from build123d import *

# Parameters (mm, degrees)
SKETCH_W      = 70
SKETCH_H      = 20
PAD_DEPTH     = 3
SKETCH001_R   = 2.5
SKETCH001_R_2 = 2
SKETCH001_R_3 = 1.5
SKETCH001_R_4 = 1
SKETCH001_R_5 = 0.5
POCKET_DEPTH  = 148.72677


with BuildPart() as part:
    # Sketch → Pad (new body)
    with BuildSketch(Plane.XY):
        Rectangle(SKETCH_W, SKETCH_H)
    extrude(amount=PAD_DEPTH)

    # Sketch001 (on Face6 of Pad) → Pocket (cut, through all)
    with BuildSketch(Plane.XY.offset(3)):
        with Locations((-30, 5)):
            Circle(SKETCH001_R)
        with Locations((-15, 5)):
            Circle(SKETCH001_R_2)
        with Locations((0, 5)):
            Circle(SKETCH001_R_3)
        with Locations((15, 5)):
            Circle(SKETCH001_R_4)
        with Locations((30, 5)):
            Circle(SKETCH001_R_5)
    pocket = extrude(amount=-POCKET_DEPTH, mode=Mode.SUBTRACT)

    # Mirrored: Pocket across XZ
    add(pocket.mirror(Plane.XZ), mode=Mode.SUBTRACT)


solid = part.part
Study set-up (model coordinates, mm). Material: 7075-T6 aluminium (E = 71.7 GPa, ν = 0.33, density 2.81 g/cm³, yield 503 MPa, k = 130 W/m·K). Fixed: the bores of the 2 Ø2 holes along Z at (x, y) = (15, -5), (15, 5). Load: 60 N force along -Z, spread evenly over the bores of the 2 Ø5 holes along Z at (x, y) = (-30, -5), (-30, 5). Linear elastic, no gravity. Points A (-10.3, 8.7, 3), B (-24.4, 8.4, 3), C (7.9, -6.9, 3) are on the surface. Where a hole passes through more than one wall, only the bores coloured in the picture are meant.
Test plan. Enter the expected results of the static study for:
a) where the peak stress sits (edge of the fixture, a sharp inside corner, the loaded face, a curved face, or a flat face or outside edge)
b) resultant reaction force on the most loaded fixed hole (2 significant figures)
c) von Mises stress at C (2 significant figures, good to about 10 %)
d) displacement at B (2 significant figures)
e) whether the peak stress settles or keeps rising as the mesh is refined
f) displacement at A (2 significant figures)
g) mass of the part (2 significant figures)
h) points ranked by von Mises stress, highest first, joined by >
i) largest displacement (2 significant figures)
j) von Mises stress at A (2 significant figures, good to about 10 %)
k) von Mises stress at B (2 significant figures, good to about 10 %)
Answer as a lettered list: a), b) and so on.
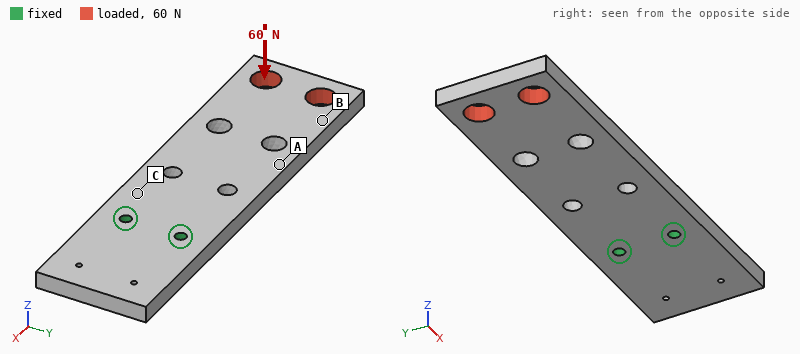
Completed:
a) edge of the fixture
b) 30 N
c) 74 MPa
d) 0.49 mm
e) keeps rising
f) 0.23 mm
g) 11 g
h) C > A > B
i) 0.71 mm
j) 43 MPa
k) 12 MPa
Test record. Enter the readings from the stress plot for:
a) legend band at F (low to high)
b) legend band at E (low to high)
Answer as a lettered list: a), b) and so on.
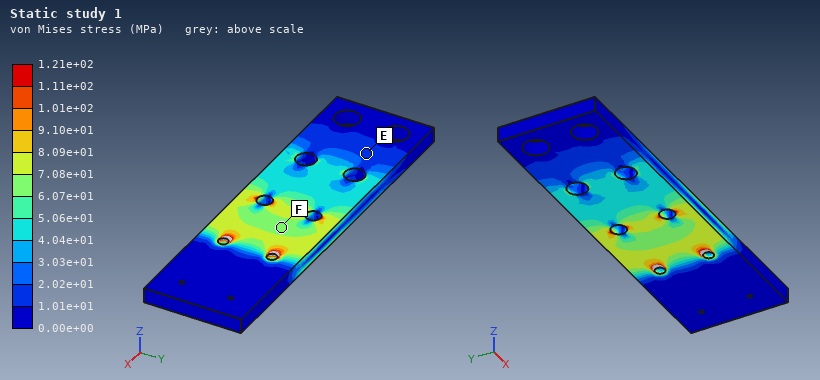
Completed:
a) 6.07e+01 to 7.08e+01 MPa
b) 1.01e+01 to 2.02e+01 MPa
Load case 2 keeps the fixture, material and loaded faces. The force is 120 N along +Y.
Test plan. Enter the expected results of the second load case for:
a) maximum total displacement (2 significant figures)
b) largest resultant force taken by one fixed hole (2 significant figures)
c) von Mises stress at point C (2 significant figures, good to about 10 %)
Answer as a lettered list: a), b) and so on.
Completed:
a) 45 µm
b) 490 N
c) 16 MPa
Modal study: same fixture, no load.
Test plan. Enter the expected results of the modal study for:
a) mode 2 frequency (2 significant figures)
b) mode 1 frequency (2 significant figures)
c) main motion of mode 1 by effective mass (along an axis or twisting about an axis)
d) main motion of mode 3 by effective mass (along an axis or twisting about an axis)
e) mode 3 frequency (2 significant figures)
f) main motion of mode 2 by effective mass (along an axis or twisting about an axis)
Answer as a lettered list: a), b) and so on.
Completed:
a) 4800 Hz
b) 1000 Hz
c) along Z
d) along Y
e) 5400 Hz
f) twisting about X
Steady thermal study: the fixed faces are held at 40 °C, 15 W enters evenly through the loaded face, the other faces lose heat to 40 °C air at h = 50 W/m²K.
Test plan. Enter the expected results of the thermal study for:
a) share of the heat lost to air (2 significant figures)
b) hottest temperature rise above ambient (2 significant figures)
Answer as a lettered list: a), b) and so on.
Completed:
a) 31 %
b) 80 K
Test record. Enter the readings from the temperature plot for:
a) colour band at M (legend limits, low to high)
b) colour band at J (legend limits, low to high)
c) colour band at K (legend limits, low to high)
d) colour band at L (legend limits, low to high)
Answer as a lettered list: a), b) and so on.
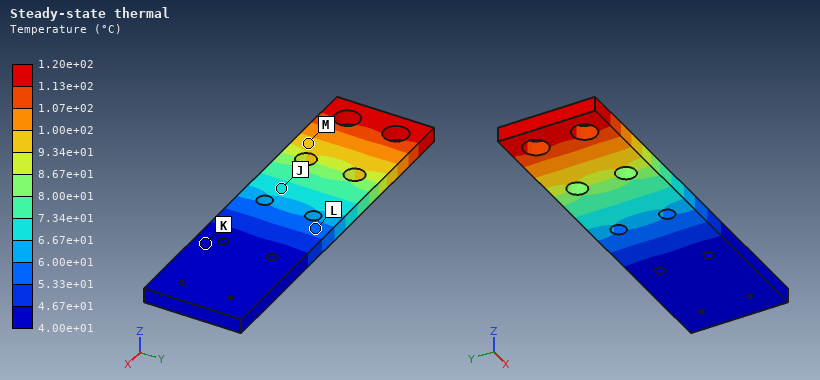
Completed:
a) 9.34e+01 to 1.00e+02 °C
b) 6.67e+01 to 7.34e+01 °C
c) 4.00e+01 to 4.67e+01 °C
d) 5.33e+01 to 6.00e+01 °C
